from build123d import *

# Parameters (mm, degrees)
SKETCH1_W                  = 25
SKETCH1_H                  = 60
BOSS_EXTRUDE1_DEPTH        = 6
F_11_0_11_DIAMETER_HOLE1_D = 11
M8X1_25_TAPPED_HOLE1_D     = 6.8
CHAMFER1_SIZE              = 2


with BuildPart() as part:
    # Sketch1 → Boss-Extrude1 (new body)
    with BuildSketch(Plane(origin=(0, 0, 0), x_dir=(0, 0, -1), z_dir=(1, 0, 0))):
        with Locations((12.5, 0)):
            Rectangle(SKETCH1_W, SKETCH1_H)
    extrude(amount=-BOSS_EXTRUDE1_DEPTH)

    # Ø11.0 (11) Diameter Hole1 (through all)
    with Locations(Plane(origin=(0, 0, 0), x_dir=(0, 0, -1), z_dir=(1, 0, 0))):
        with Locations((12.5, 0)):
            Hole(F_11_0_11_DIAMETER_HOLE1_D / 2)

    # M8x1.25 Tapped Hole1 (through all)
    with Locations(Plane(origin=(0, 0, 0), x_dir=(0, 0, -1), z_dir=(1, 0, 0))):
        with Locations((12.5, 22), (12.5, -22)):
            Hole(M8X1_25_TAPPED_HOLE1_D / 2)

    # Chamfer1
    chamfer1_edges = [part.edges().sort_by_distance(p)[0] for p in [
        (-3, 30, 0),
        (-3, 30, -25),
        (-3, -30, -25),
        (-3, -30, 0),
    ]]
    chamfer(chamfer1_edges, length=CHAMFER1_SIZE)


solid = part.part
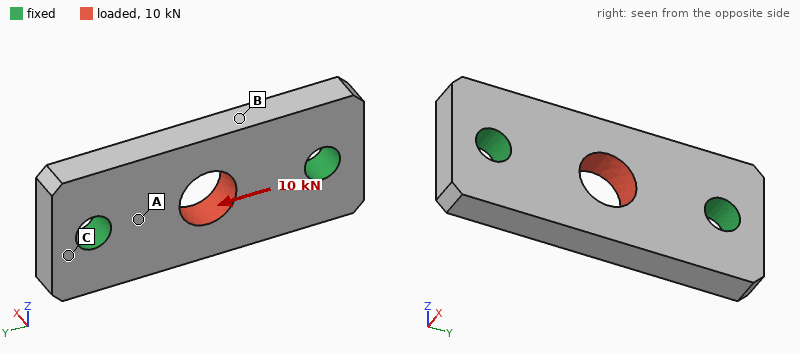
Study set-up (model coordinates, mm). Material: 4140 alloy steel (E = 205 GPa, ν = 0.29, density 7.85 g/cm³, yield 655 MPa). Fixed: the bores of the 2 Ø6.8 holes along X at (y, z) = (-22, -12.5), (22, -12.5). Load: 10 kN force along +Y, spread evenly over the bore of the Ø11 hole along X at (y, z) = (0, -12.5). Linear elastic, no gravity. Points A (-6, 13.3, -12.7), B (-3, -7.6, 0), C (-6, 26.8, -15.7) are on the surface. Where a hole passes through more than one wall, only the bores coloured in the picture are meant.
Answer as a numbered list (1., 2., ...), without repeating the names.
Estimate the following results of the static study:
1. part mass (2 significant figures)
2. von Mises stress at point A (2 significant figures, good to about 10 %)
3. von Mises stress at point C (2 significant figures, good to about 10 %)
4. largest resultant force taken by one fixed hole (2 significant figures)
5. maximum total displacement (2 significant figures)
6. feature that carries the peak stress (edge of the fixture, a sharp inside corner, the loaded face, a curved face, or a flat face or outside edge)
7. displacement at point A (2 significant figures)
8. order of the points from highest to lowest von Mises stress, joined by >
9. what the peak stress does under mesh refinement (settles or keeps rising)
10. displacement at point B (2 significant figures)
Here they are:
1. 62 g
2. 63 MPa
3. 18 MPa
4. 5.0 kN
5. 4.7 µm
6. edge of the fixture
7. 1.7 µm
8. A > C > B
9. keeps rising
10. 2.7 µm
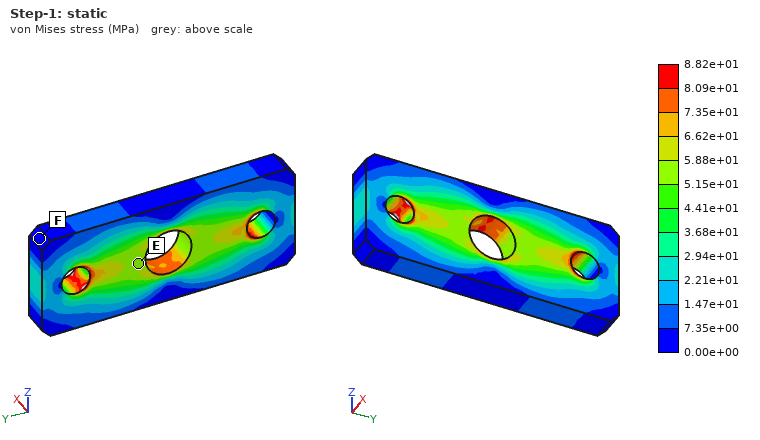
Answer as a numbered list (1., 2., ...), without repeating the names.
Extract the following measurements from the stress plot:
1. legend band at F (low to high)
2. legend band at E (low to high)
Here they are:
1. 0.00e+00 to 7.35e+00 MPa
2. 5.15e+01 to 5.88e+01 MPa
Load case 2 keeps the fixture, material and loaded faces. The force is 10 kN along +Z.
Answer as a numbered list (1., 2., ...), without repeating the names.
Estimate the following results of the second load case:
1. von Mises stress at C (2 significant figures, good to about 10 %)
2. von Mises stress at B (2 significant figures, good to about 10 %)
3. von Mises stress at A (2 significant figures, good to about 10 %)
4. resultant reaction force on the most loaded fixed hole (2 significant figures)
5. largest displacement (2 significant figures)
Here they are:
1. 25 MPa
2. 72 MPa
3. 84 MPa
4. 5.0 kN
5. 15 µm
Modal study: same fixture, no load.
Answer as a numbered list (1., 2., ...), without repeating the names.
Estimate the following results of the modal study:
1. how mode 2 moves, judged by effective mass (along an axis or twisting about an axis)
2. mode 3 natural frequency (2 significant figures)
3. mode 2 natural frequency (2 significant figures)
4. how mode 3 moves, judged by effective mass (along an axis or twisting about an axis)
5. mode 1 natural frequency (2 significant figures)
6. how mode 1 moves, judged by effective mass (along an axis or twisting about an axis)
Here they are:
1. twisting about Y
2. 29 kHz
3. 17 kHz
4. along Z
5. 16 kHz
6. along X
